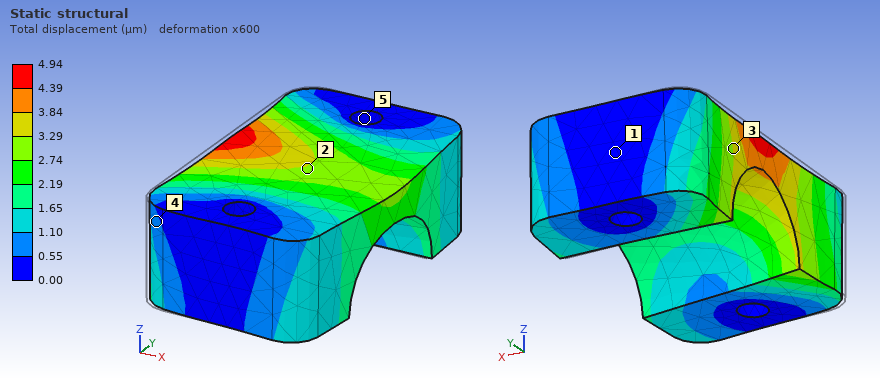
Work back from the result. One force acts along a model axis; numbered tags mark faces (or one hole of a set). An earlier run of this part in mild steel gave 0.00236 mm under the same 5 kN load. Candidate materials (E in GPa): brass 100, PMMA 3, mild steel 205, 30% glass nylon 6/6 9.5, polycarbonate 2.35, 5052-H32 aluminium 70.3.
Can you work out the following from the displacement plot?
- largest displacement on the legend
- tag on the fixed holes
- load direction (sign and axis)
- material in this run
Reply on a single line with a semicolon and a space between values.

4.94 µm; 5; +X; brass
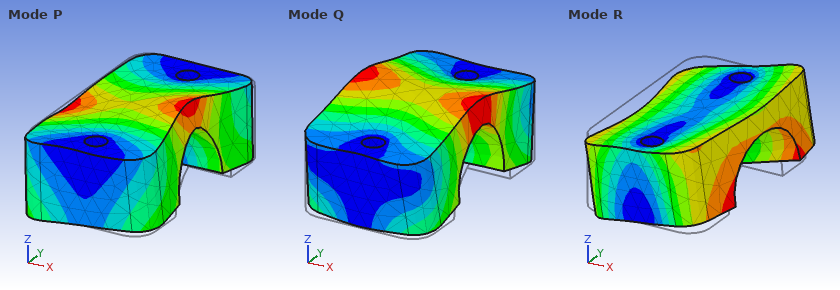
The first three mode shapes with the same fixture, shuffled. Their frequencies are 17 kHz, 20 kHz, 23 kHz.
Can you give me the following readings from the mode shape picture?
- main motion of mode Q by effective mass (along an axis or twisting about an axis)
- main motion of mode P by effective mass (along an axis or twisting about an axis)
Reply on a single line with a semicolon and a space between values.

along Z; along X
